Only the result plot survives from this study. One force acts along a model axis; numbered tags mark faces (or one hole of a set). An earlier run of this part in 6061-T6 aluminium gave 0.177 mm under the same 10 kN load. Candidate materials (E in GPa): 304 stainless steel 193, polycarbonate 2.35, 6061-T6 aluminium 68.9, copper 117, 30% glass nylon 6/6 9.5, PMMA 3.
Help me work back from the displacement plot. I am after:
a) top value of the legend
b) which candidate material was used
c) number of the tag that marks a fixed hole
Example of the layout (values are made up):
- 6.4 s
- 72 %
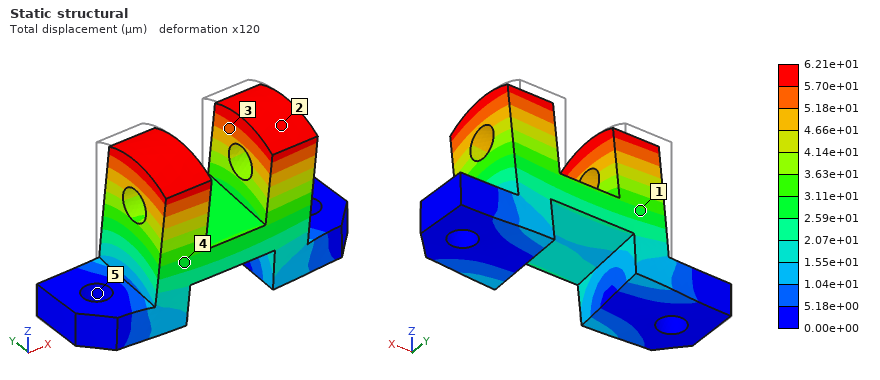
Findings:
- 6.21e+01 µm
- 304 stainless steel
- 5
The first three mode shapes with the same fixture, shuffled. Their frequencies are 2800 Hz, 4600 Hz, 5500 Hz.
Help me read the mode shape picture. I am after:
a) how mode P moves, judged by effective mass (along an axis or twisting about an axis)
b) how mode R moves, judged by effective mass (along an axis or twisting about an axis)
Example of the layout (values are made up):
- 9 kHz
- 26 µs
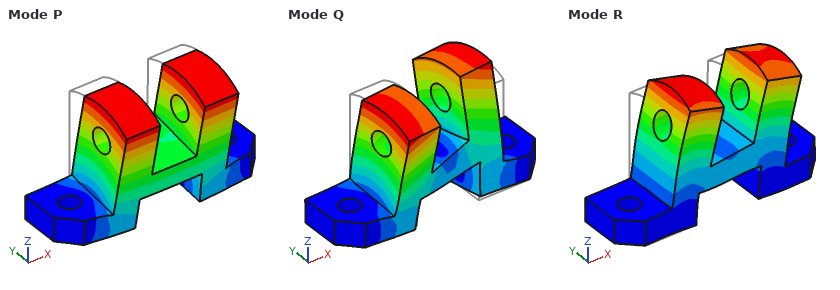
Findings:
- along Y
- along X
